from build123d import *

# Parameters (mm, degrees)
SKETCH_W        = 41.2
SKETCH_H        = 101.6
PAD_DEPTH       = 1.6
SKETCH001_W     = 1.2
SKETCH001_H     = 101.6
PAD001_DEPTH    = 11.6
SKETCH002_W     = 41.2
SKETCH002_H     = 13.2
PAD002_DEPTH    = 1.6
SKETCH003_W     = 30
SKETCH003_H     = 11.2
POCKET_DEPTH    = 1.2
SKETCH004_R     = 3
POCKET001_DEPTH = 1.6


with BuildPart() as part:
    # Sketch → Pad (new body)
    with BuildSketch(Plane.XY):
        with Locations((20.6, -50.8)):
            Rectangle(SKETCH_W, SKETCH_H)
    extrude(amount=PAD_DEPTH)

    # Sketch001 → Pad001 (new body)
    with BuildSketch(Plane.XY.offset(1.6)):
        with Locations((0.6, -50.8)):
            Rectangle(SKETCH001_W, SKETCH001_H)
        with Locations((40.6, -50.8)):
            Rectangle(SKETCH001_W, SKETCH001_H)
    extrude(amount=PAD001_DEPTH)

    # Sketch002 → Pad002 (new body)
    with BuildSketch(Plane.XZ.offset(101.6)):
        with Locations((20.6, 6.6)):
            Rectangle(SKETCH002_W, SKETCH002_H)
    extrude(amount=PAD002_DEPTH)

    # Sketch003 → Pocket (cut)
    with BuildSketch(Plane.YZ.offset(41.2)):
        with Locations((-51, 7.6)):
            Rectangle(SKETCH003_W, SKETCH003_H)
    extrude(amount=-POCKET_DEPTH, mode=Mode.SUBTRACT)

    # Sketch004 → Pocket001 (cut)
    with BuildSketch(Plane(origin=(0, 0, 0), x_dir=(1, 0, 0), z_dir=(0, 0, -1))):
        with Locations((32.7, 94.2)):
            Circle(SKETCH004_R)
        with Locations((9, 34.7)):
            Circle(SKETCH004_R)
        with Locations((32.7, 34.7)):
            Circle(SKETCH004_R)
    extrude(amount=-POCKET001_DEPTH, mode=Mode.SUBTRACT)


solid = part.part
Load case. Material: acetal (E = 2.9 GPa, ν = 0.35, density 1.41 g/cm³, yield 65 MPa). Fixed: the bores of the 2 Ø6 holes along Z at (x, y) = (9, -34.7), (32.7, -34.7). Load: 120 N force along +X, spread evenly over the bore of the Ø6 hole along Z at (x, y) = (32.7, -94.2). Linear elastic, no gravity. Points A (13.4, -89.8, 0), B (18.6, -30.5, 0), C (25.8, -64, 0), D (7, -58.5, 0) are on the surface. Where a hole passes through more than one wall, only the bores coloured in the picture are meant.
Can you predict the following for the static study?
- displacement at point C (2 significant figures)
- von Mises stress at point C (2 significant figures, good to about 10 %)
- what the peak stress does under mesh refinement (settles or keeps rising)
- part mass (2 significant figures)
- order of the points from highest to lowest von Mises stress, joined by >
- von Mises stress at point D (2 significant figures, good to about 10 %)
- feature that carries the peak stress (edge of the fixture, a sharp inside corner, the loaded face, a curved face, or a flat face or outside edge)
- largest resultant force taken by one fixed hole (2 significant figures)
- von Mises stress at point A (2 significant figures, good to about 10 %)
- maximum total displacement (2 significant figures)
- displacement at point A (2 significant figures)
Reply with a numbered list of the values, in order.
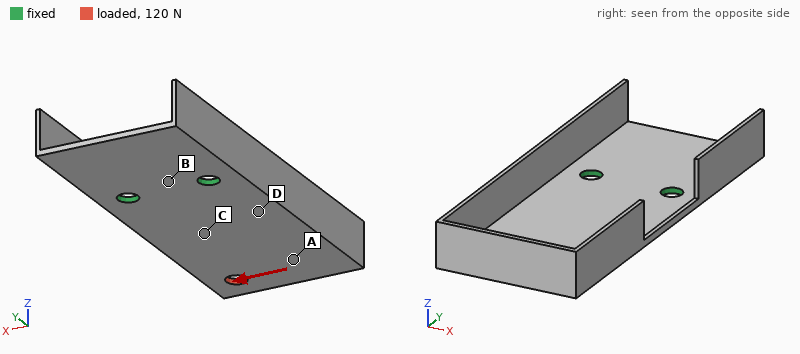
1. 0.19 mm
2. 4.6 MPa
3. keeps rising
4. 14 g
5. D > C > A > B
6. 6.4 MPa
7. edge of the fixture
8. 270 N
9. 2.6 MPa
10. 0.75 mm
11. 0.50 mm
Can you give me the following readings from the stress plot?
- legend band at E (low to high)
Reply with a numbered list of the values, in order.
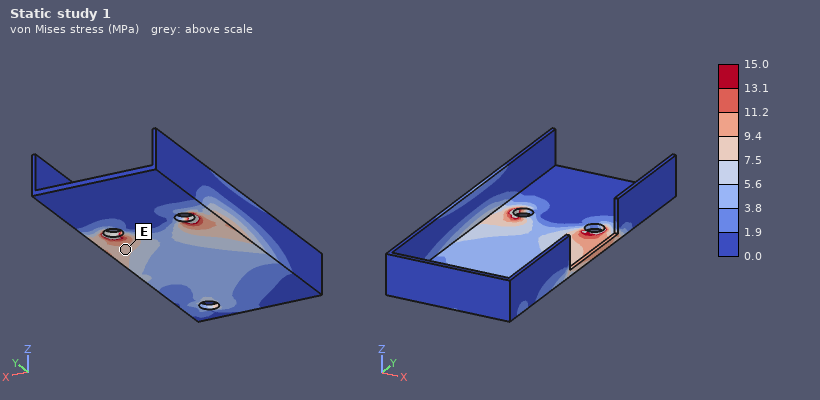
1. 7.5 to 9.4 MPa
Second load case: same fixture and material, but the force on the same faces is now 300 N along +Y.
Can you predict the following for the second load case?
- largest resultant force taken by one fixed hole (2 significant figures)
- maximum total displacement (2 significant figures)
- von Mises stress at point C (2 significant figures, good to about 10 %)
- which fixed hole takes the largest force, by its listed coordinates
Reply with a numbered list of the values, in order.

1. 290 N
2. 0.38 mm
3. 6.2 MPa
4. (32.7, -34.7)
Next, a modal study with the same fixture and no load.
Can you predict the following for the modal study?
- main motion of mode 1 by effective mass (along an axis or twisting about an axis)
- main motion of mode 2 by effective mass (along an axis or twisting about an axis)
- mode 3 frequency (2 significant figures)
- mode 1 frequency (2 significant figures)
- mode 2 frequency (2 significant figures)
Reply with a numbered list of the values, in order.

1. along Z
2. twisting about Y
3. 500 Hz
4. 120 Hz
5. 240 Hz
